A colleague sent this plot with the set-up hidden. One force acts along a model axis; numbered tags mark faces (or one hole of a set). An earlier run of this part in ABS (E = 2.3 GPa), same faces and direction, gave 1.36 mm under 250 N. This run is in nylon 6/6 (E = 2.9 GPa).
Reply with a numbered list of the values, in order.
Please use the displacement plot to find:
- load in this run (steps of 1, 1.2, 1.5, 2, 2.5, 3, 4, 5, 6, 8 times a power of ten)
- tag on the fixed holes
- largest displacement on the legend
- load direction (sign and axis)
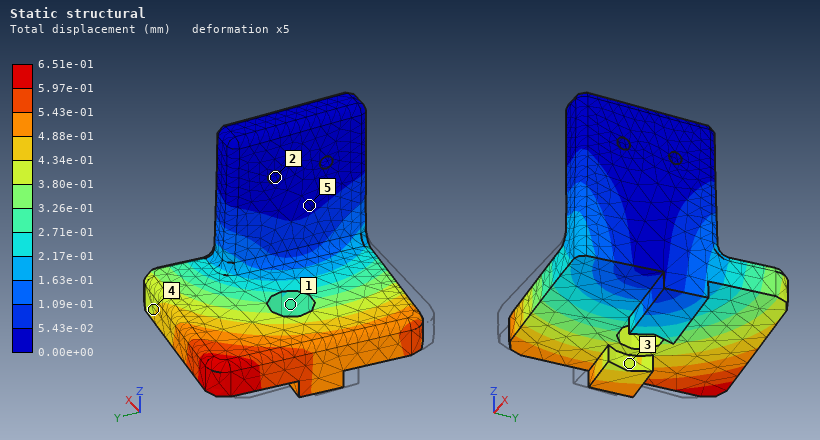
1. 150 N
2. 2
3. 6.51e-01 mm
4. +Y
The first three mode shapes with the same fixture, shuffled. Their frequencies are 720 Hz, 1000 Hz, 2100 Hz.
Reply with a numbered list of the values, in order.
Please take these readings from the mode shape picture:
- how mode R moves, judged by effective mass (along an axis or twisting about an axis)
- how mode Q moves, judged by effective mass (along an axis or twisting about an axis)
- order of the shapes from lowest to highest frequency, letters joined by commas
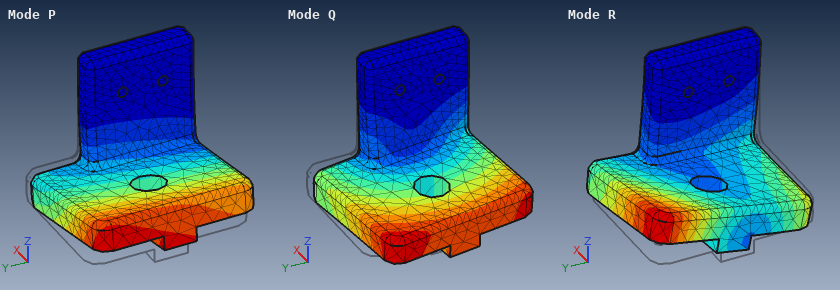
1. along X
2. along Y
3. P, Q, R
